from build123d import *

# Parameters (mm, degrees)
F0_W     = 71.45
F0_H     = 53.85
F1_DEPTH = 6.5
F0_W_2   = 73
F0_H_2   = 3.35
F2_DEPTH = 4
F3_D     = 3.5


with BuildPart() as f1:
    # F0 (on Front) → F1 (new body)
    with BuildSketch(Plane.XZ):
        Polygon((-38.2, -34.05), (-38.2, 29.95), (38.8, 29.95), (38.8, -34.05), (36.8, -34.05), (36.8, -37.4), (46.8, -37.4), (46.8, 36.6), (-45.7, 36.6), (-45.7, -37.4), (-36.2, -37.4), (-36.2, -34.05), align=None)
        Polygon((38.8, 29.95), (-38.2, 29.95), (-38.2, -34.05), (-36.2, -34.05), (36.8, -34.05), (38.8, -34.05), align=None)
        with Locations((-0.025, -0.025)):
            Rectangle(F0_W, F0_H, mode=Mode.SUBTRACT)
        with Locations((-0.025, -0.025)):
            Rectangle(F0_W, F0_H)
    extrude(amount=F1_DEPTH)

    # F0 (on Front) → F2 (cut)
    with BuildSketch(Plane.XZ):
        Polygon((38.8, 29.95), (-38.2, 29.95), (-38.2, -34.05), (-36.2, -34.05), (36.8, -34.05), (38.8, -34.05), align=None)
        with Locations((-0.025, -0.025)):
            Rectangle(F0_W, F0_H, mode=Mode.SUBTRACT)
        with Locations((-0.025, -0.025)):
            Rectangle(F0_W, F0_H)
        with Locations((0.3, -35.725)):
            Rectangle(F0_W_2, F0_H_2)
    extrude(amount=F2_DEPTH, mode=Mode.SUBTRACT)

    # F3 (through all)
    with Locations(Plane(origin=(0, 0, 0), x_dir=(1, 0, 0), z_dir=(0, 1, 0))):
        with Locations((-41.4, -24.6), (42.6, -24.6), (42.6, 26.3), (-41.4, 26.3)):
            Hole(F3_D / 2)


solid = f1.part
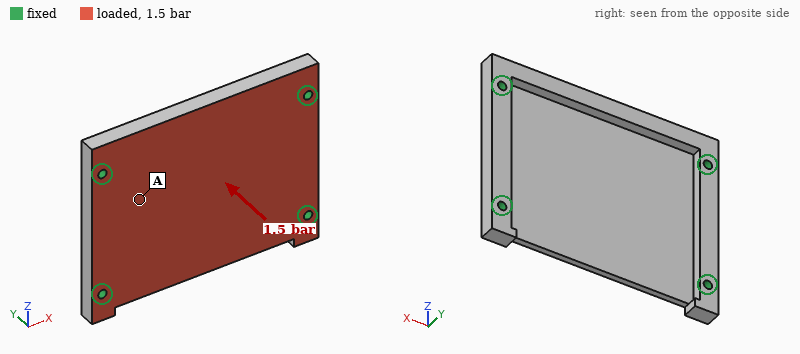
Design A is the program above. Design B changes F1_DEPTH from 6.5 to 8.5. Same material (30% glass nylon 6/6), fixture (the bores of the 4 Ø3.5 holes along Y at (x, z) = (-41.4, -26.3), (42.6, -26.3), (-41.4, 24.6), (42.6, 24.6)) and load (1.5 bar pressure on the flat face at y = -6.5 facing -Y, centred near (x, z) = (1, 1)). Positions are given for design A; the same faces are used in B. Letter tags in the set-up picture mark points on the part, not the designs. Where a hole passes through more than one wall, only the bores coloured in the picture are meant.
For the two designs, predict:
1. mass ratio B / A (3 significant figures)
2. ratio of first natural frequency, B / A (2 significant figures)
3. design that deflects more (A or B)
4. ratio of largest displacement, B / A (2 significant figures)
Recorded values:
1.57
1.5
A
0.21
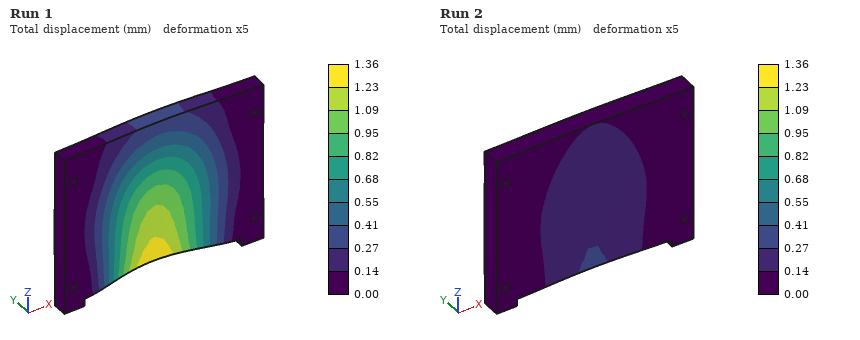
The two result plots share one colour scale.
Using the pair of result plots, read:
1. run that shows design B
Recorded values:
Run 2
